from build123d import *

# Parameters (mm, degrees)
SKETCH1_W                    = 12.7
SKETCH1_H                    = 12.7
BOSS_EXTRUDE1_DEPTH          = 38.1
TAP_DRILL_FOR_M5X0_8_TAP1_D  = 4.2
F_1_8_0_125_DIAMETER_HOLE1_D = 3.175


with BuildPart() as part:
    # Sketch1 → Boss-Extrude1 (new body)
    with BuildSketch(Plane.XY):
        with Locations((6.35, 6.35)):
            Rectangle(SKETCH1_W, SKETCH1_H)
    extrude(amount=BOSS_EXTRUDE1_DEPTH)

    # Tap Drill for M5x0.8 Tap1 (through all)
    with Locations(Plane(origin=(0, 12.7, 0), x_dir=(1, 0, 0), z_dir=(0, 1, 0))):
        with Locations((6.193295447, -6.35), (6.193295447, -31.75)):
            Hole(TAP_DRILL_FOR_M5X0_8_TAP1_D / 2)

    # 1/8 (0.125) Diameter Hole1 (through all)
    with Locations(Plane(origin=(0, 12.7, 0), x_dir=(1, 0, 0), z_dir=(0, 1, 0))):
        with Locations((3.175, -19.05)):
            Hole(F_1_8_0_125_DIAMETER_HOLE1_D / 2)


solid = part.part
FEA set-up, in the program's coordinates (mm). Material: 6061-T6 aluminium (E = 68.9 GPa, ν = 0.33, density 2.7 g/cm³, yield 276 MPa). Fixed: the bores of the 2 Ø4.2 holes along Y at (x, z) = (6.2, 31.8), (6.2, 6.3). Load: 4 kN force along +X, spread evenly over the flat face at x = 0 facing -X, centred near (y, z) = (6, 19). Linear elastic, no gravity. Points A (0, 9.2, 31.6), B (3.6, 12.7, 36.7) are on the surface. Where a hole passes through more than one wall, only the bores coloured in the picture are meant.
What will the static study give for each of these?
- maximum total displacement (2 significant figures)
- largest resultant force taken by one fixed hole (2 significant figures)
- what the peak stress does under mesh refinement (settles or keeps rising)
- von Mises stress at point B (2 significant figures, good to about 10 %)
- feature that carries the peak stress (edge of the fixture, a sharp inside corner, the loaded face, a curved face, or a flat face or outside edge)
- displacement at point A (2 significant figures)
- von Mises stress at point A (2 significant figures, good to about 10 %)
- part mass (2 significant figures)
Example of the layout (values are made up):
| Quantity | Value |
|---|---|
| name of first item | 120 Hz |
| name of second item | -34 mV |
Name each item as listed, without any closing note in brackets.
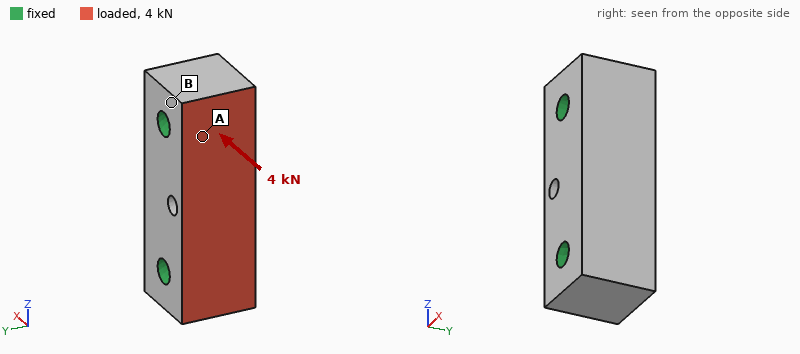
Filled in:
| Quantity | Value |
|---|---|
| maximum total displacement | 4.2 µm |
| largest resultant force taken by one fixed hole | 2.0 kN |
| what the peak stress does under mesh refinement | keeps rising |
| von Mises stress at point B | 5.8 MPa |
| feature that carries the peak stress | edge of the fixture |
| displacement at point A | 0.89 µm |
| von Mises stress at point A | 17 MPa |
| part mass | 15 g |
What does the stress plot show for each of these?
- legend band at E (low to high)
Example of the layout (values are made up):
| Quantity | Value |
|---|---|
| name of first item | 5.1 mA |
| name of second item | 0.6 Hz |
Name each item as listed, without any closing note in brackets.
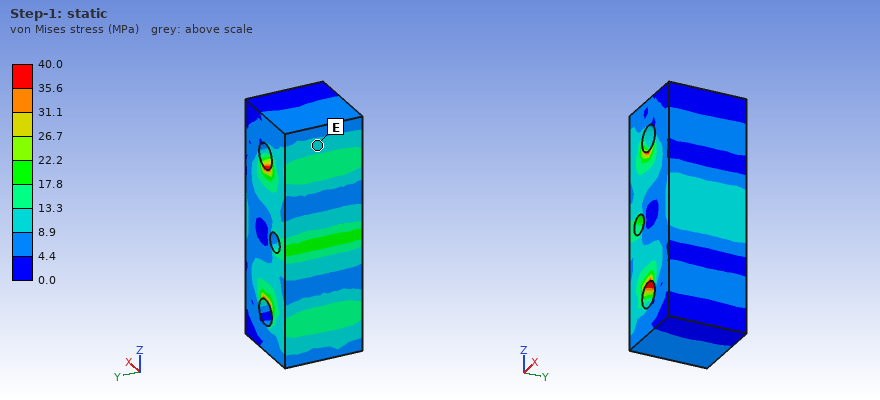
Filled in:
| Quantity | Value |
|---|---|
| legend band at E | 8.9 to 13.3 MPa |
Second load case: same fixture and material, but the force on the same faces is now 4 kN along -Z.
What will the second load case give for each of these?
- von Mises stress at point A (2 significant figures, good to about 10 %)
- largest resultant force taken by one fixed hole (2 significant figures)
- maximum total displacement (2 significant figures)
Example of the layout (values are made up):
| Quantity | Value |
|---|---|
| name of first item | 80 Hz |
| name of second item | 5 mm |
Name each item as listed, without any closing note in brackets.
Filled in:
| Quantity | Value |
|---|---|
| von Mises stress at point A | 16 MPa |
| largest resultant force taken by one fixed hole | 2.1 kN |
| maximum total displacement | 4.5 µm |
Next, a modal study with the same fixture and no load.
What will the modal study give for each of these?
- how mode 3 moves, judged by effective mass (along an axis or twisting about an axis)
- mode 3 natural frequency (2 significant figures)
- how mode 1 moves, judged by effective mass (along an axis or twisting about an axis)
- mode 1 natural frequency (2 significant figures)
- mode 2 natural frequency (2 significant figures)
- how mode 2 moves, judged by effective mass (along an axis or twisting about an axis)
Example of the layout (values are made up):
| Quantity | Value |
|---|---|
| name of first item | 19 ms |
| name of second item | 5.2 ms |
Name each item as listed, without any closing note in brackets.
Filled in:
| Quantity | Value |
|---|---|
| how mode 3 moves, judged by effective mass | twisting about Z |
| mode 3 natural frequency | 59 kHz |
| how mode 1 moves, judged by effective mass | along X |
| mode 1 natural frequency | 46 kHz |
| mode 2 natural frequency | 52 kHz |
| how mode 2 moves, judged by effective mass | along Y |
